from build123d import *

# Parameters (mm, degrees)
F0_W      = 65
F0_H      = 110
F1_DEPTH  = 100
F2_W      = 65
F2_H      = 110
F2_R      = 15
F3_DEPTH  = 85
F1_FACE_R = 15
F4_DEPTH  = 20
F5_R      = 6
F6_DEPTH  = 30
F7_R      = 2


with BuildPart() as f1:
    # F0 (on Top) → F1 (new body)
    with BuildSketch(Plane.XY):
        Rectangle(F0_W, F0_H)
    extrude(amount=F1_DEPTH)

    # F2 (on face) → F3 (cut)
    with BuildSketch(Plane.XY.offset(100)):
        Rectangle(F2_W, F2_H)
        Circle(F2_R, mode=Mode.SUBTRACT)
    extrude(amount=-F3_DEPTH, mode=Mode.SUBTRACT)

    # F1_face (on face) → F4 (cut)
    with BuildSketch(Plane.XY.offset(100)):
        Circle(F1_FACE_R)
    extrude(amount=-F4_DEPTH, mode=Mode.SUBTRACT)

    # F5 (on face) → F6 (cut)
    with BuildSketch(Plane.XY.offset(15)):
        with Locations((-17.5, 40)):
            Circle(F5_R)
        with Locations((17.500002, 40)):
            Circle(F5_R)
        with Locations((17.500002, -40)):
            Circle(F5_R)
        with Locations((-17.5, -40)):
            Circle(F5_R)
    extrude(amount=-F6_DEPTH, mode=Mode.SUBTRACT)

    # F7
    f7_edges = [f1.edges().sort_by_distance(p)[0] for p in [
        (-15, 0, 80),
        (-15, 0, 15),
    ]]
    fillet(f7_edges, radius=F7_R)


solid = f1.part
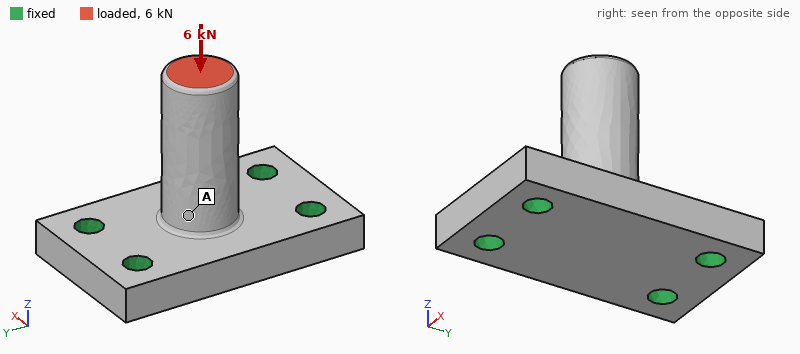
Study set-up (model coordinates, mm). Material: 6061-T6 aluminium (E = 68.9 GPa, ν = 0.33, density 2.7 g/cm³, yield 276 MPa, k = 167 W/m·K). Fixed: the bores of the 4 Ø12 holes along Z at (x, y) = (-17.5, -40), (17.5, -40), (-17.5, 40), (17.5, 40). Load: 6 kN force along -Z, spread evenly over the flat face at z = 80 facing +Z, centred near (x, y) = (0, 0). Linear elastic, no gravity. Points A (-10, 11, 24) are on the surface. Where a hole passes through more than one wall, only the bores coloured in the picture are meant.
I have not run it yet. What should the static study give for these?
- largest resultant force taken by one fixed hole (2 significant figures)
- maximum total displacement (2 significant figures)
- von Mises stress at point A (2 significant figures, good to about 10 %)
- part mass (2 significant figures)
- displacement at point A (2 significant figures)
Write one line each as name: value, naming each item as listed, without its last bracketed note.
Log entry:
largest resultant force taken by one fixed hole: 1.5 kN
maximum total displacement: 19 µm
von Mises stress at point A: 8.0 MPa
part mass: 400 g
displacement at point A: 12 µm
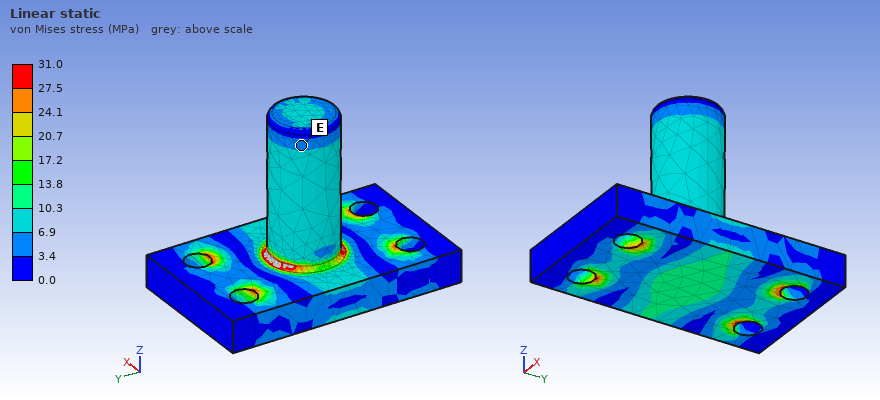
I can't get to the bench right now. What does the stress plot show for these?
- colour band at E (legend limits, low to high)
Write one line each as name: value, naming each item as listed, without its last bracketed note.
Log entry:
colour band at E: 3.4 to 6.9 MPa
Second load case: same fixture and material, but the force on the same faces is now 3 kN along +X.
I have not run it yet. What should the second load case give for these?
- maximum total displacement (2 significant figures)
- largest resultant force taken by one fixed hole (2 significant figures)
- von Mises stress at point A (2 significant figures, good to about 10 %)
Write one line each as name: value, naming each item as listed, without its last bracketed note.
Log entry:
maximum total displacement: 0.21 mm
largest resultant force taken by one fixed hole: 2.7 kN
von Mises stress at point A: 40 MPa
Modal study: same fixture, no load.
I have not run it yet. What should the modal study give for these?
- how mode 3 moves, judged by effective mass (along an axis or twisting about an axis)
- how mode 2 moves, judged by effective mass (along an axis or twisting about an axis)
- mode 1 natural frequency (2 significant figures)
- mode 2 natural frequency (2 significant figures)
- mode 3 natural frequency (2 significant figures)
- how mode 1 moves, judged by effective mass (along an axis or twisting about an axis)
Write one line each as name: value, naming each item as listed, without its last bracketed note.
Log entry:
how mode 3 moves, judged by effective mass: along Z
how mode 2 moves, judged by effective mass: along Y
mode 1 natural frequency: 3100 Hz
mode 2 natural frequency: 3500 Hz
mode 3 natural frequency: 7700 Hz
how mode 1 moves, judged by effective mass: along X
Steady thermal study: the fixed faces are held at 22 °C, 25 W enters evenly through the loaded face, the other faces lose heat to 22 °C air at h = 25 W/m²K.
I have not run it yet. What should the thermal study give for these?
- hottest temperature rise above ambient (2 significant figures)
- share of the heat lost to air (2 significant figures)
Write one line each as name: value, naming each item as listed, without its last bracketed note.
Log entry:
hottest temperature rise above ambient: 17 K
share of the heat lost to air: 7.4 %
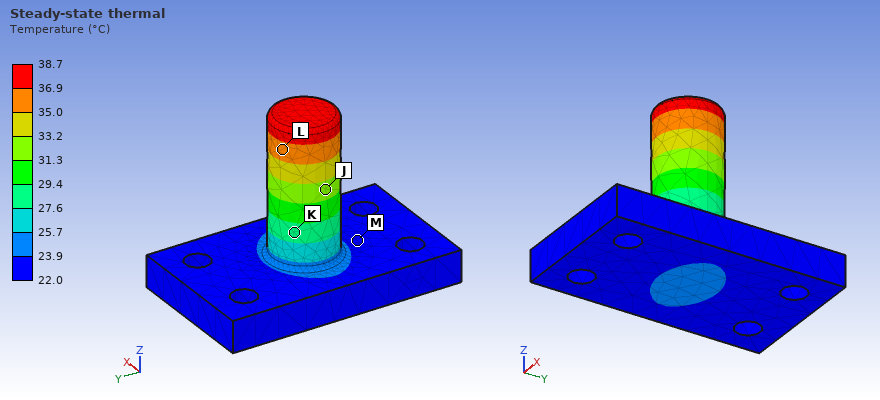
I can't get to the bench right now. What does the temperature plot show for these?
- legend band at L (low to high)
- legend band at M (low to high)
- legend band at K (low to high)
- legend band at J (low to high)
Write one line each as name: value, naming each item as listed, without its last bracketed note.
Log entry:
legend band at L: 35.0 to 36.9 °C
legend band at M: 22.0 to 23.9 °C
legend band at K: 27.6 to 29.4 °C
legend band at J: 31.3 to 33.2 °C
